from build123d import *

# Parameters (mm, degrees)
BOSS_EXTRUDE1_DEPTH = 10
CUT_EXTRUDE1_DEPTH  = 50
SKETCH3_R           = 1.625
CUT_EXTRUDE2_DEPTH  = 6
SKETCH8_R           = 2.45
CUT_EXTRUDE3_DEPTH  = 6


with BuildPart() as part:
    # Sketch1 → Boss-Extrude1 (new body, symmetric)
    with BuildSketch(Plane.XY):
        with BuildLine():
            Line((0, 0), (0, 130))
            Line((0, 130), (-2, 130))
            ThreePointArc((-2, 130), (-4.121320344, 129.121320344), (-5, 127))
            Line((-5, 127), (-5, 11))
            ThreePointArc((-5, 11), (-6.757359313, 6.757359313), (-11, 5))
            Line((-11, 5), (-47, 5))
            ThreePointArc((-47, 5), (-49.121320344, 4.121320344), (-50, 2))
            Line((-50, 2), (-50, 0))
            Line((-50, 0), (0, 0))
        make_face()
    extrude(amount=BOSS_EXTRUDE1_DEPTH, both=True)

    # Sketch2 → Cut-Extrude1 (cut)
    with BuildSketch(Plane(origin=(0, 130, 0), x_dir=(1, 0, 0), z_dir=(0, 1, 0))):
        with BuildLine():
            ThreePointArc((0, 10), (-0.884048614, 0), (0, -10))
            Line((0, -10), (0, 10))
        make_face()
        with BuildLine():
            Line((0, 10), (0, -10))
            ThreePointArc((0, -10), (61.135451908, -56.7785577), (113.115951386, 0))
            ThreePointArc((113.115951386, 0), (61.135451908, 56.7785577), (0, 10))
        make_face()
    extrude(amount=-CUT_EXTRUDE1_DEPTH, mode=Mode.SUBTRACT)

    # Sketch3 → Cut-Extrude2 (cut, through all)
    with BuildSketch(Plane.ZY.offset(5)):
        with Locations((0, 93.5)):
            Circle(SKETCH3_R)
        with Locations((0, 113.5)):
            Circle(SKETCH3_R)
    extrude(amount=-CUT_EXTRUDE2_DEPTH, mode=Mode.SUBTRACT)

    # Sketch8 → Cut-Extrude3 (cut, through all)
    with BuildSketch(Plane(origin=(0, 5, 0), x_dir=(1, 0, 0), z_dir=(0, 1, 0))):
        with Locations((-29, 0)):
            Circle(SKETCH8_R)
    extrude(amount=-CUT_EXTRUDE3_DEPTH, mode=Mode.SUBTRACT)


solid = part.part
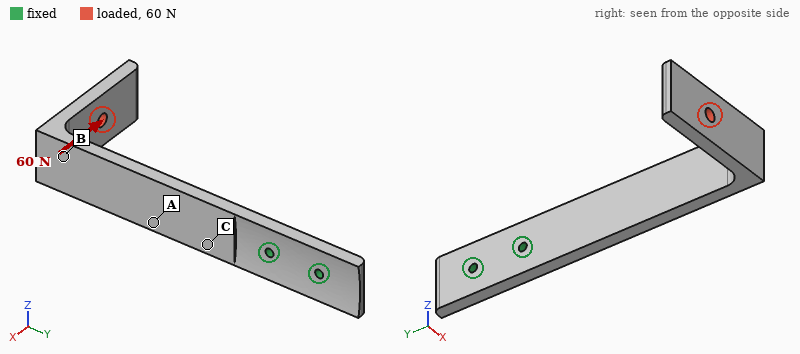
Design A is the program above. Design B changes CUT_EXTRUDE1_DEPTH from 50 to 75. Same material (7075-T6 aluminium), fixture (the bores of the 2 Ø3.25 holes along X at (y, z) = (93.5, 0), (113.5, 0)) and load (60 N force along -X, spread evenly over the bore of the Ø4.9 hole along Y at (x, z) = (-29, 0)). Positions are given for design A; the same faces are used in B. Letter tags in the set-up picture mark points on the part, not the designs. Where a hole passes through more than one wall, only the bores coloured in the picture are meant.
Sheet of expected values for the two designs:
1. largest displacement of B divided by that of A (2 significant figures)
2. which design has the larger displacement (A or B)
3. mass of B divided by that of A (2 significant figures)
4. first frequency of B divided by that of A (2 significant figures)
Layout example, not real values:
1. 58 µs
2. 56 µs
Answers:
1. 1.1
2. B
3. 0.98
4. 0.94
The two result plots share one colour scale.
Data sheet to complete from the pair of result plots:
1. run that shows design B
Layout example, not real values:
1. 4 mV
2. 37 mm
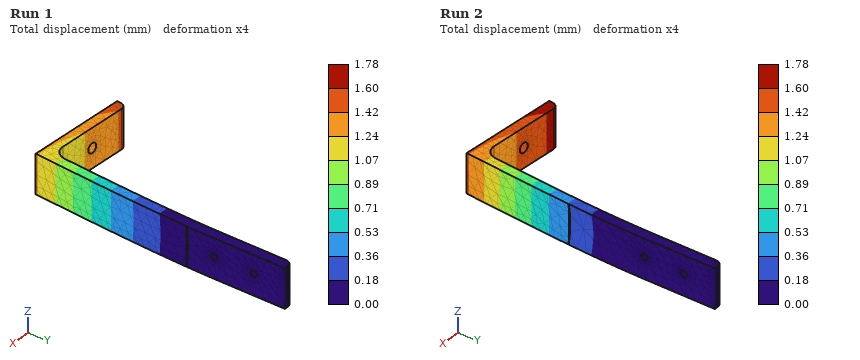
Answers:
1. Run 2
